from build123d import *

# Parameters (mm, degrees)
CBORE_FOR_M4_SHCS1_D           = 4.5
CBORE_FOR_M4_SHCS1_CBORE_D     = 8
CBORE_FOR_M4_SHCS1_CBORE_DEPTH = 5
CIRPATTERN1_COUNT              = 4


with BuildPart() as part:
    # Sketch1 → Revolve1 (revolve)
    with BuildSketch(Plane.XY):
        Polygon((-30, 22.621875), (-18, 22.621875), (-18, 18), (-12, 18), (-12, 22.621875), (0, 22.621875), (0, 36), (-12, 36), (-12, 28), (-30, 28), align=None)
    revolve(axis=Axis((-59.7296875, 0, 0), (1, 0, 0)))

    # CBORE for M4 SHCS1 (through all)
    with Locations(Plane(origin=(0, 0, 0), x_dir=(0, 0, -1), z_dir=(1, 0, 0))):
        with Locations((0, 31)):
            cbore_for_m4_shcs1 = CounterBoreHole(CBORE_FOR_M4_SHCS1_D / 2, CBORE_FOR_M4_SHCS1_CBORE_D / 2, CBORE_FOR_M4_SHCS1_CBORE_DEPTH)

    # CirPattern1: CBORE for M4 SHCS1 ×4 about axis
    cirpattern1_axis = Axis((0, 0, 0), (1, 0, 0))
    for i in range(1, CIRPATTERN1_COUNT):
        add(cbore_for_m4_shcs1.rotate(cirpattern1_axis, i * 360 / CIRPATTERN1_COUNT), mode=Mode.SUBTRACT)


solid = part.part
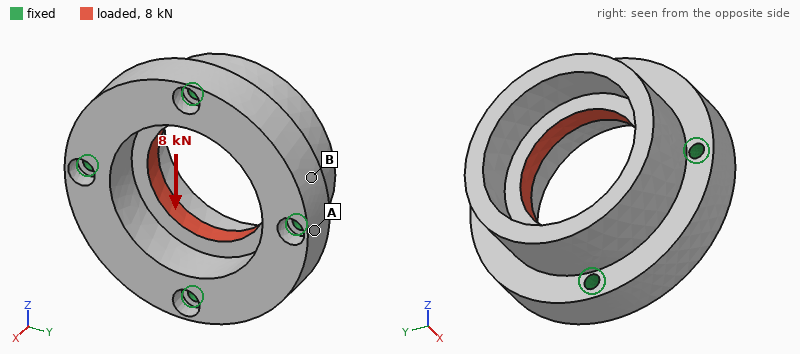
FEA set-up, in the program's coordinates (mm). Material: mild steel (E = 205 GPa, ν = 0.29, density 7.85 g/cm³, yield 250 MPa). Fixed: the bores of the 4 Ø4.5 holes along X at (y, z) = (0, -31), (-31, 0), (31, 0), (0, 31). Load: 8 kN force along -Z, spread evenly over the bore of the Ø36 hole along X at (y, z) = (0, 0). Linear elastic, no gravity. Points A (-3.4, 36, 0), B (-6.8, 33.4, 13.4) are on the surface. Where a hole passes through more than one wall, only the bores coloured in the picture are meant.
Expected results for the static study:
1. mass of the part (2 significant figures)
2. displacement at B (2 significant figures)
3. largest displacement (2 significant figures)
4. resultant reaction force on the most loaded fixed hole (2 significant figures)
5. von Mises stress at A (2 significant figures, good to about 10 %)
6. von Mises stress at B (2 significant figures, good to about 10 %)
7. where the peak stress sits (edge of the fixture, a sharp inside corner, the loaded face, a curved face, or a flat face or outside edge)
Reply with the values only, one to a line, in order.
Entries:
370 g
0.75 µm
2.7 µm
2.3 kN
4.5 MPa
8.3 MPa
edge of the fixture
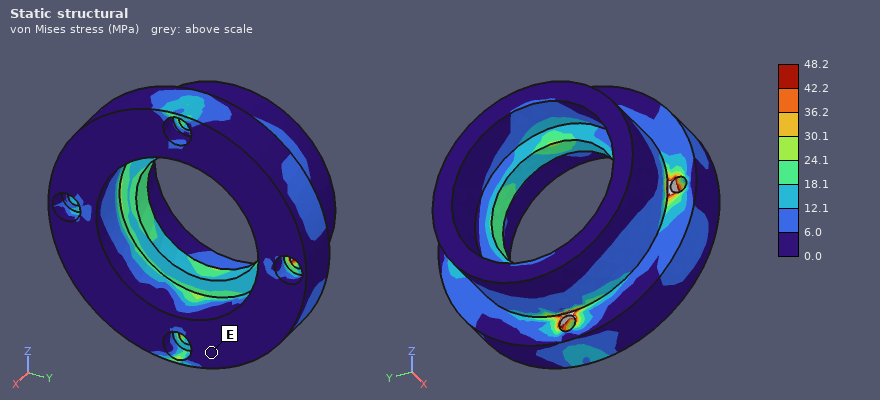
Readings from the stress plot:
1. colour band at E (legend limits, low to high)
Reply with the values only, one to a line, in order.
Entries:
0.0 to 6.0 MPa
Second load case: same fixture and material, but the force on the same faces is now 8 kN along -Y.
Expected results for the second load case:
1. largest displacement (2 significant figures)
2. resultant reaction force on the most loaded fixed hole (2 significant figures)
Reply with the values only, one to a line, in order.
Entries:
2.7 µm
2.3 kN
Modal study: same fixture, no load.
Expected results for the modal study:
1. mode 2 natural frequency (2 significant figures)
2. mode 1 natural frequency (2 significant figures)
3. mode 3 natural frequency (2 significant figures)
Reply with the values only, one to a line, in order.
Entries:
16 kHz
12 kHz
16 kHz
